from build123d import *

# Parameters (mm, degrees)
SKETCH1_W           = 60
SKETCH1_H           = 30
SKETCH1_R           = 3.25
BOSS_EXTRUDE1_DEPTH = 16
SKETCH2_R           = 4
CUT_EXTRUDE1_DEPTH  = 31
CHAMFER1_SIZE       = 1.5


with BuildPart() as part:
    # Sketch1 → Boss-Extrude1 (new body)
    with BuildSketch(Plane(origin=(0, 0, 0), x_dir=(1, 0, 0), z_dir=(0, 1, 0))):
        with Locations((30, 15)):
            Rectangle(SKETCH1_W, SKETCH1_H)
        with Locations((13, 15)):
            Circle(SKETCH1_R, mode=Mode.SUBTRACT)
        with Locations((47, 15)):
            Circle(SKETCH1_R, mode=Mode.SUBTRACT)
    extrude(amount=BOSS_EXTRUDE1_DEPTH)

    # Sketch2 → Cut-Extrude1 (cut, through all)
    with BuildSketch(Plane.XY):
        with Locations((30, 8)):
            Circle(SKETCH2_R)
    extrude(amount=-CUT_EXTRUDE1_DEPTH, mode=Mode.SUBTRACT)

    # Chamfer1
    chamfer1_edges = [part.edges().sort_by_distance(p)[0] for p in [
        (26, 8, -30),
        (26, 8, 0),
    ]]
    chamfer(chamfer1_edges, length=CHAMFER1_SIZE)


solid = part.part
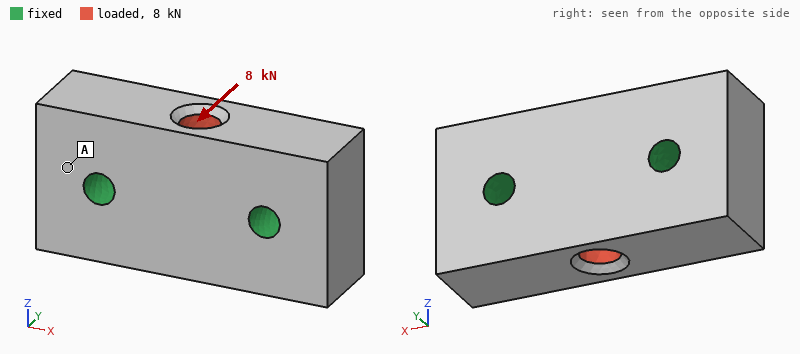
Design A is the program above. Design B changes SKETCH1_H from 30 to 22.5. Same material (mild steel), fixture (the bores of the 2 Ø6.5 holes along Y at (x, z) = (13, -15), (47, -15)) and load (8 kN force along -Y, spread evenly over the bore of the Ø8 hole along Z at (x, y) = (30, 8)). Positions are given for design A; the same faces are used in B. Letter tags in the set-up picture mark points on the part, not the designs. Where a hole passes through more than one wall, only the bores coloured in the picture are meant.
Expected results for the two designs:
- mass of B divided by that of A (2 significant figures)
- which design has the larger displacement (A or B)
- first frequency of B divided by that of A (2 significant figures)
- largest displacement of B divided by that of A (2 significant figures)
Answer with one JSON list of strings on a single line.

["0.74", "B", "1.1", "1.1"]
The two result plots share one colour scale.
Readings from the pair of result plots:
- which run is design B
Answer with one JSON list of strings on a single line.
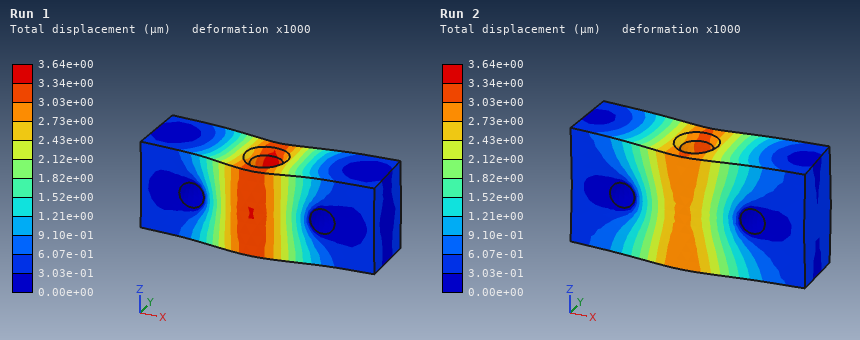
["Run 1"]
